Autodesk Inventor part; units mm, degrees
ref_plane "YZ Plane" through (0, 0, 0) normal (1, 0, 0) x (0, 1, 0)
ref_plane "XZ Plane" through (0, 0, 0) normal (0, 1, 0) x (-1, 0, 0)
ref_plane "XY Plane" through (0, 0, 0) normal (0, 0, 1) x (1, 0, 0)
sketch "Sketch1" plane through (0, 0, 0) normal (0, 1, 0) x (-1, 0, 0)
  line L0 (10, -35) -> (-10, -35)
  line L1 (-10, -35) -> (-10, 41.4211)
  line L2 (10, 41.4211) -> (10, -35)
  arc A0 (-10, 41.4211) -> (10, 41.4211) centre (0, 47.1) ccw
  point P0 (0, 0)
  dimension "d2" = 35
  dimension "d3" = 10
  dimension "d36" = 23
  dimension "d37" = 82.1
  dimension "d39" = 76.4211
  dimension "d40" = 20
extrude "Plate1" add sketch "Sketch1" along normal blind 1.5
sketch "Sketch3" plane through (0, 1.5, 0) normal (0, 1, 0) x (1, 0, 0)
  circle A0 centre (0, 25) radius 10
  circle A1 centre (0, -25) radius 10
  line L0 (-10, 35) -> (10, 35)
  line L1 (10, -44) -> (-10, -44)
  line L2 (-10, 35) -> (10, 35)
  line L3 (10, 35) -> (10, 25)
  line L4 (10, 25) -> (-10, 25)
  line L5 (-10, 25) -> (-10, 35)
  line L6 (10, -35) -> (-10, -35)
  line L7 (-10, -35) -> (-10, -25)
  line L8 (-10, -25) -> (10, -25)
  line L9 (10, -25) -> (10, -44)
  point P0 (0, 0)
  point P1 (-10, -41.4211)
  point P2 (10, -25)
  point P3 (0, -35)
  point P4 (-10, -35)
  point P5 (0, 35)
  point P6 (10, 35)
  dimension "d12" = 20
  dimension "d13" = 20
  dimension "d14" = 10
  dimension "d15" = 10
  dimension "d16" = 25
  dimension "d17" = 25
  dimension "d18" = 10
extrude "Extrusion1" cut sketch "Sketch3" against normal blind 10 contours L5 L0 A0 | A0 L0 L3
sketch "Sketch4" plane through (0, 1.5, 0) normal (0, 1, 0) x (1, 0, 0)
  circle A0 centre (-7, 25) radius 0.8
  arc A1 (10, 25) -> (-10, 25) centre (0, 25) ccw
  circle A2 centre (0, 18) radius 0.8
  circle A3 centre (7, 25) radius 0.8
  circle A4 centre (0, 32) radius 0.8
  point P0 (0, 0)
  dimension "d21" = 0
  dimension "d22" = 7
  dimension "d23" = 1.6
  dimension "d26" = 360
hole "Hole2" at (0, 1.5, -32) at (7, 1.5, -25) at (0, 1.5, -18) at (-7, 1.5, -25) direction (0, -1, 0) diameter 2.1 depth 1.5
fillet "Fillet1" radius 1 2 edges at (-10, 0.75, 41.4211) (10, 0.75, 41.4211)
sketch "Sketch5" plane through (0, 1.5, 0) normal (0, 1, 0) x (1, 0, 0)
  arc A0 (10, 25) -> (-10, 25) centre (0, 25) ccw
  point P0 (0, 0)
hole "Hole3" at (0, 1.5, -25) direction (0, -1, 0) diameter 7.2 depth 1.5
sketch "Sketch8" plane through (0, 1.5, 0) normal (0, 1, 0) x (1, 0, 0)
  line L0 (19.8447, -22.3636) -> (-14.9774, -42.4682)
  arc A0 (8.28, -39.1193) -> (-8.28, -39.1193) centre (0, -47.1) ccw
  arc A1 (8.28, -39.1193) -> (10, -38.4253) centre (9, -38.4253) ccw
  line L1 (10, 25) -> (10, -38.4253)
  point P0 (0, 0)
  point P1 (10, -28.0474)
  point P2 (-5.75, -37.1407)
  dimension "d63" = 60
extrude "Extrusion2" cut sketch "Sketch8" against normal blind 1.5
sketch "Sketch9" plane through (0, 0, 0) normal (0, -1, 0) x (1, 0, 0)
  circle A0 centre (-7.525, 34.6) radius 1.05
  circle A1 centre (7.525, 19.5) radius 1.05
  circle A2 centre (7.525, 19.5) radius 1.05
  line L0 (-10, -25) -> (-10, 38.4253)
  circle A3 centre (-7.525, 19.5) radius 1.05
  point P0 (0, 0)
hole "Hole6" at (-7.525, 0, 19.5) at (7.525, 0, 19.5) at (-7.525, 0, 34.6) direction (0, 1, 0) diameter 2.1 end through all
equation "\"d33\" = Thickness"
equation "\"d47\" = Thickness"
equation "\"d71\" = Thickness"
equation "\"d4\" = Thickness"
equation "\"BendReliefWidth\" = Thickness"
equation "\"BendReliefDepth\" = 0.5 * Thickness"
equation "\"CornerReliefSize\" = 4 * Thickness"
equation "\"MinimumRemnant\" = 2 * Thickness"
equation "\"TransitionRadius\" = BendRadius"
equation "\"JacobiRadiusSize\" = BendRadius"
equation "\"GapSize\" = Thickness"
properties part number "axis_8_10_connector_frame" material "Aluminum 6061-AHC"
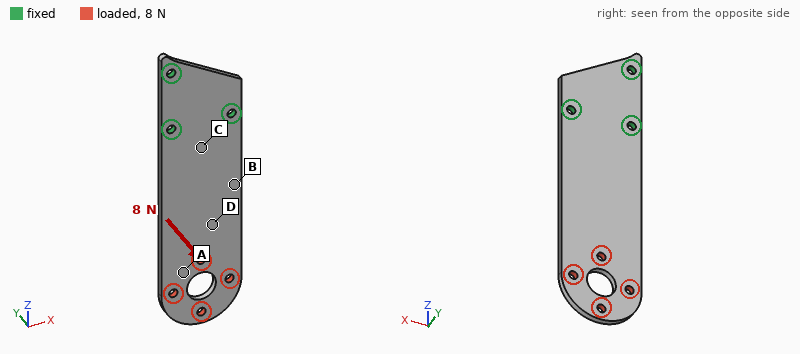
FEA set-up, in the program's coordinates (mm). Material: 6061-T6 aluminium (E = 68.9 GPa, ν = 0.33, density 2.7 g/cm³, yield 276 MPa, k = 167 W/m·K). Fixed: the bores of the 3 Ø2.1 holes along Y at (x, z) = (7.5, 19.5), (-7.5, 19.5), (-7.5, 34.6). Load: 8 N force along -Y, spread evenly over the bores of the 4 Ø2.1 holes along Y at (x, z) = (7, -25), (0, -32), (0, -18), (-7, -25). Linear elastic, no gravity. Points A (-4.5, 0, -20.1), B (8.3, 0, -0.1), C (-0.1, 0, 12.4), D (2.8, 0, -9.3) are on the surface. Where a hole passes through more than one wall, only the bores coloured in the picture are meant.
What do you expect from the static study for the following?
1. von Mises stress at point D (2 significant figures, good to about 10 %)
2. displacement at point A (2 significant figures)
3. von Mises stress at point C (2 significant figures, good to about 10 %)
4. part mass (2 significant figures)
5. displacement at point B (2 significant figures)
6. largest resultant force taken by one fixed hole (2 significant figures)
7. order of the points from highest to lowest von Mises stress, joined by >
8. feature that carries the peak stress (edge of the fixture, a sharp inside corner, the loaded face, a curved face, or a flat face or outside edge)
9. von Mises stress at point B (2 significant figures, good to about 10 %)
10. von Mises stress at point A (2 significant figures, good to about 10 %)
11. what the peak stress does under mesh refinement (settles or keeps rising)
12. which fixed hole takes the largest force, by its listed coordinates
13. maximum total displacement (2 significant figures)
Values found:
17 MPa
0.50 mm
37 MPa
5.1 g
0.15 mm
6.9 N
C > B > D > A
edge of the fixture
27 MPa
7.4 MPa
keeps rising
(-7.5, 19.5)
0.81 mm
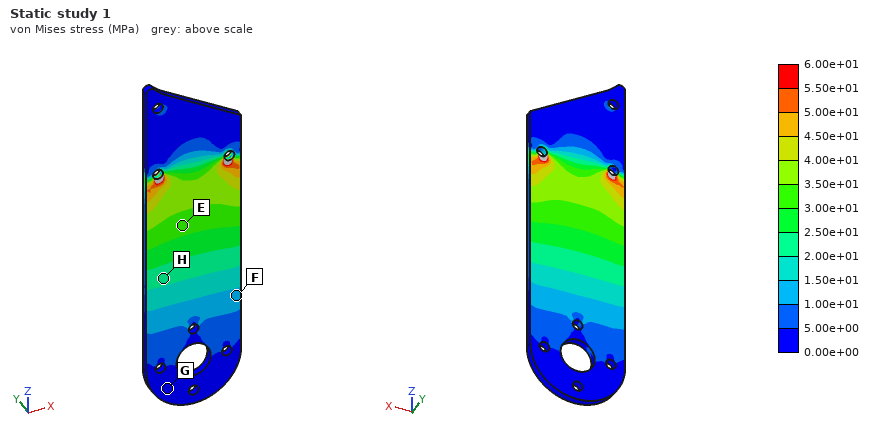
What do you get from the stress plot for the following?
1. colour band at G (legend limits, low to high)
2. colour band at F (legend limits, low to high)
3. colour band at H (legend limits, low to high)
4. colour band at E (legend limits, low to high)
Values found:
0.00e+00 to 5.00e+00 MPa
1.00e+01 to 1.50e+01 MPa
2.00e+01 to 2.50e+01 MPa
3.00e+01 to 3.50e+01 MPa
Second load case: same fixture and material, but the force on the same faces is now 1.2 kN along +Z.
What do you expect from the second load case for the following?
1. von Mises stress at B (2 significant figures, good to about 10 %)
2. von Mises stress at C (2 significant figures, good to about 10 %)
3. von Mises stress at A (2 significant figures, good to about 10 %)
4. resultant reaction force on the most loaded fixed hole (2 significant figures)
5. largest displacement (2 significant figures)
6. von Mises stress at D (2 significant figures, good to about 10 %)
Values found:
40 MPa
31 MPa
45 MPa
570 N
34 µm
40 MPa
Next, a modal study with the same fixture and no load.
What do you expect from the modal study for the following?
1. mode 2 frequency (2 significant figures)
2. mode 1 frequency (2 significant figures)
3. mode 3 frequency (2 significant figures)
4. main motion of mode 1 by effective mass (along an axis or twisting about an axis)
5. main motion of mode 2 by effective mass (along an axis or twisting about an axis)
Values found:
2600 Hz
480 Hz
2800 Hz
along Y
twisting about Z
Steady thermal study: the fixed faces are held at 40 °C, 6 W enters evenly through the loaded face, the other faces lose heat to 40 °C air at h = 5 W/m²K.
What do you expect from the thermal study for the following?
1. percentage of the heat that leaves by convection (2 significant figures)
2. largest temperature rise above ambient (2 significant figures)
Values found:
5.6 %
58 K
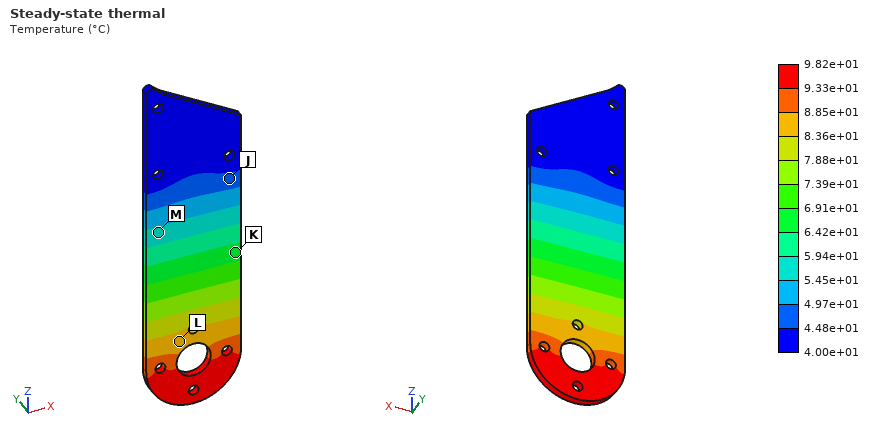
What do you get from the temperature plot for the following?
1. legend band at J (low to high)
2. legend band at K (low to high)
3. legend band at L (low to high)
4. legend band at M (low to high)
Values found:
4.48e+01 to 4.97e+01 °C
6.42e+01 to 6.91e+01 °C
8.36e+01 to 8.85e+01 °C
5.45e+01 to 5.94e+01 °C
